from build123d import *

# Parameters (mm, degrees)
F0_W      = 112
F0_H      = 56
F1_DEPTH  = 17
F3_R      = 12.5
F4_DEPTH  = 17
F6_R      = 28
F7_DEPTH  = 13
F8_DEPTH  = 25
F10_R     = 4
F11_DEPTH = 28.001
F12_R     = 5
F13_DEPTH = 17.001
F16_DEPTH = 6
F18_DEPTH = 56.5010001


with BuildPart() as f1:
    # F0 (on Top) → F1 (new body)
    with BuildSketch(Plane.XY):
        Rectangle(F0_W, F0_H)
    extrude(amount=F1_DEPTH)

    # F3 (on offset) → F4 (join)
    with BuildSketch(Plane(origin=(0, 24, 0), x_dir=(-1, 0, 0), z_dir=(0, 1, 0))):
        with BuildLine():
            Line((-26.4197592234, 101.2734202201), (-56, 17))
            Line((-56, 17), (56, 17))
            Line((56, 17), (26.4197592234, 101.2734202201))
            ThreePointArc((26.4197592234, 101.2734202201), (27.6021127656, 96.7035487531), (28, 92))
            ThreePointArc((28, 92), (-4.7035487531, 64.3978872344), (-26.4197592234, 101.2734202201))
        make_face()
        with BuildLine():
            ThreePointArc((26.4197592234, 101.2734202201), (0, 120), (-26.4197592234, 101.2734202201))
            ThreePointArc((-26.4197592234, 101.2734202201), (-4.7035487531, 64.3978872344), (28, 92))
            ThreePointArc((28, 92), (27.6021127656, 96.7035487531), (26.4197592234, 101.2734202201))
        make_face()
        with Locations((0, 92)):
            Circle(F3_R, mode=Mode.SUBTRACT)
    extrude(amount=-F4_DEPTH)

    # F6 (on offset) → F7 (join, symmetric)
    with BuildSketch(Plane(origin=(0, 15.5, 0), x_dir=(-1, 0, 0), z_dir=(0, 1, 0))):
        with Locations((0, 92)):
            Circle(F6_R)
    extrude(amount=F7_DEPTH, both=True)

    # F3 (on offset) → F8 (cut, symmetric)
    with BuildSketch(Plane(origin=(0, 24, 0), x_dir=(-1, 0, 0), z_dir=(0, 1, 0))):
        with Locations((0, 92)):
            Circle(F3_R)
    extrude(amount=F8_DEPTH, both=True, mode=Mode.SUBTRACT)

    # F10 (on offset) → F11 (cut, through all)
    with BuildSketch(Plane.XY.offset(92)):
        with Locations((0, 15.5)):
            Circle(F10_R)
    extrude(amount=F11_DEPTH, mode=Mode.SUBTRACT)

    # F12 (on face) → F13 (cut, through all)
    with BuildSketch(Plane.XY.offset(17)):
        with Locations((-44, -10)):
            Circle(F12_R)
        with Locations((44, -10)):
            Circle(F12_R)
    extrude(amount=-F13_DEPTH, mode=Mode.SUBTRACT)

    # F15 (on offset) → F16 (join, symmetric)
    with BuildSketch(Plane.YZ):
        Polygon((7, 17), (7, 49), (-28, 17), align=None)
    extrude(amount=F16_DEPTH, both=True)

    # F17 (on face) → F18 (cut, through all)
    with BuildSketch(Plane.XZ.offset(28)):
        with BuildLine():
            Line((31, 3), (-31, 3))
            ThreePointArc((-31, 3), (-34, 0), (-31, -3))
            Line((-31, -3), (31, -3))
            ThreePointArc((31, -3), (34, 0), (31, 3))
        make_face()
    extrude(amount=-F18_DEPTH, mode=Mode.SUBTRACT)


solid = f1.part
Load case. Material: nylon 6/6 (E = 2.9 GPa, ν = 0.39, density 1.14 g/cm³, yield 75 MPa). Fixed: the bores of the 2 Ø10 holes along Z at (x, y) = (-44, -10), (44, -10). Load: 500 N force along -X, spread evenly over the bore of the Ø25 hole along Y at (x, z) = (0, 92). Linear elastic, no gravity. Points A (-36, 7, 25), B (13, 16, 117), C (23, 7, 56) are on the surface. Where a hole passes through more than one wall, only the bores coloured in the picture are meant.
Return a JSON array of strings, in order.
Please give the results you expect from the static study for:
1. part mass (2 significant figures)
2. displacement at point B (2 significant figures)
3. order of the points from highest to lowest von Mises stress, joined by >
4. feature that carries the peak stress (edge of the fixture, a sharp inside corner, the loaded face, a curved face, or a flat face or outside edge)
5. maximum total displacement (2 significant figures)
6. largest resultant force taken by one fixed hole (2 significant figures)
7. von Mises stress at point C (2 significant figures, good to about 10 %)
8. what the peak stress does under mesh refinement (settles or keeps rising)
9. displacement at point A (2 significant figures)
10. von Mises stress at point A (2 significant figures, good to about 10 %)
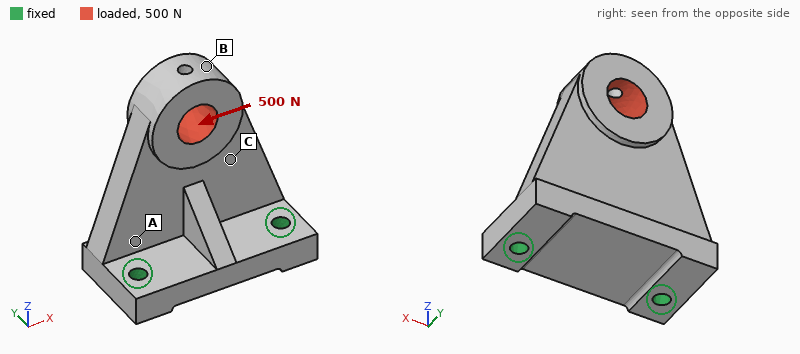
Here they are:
["270 g", "0.18 mm", "A > C > B", "edge of the fixture", "0.19 mm", "550 N", "0.94 MPa", "keeps rising", "0.044 mm", "2.1 MPa"]
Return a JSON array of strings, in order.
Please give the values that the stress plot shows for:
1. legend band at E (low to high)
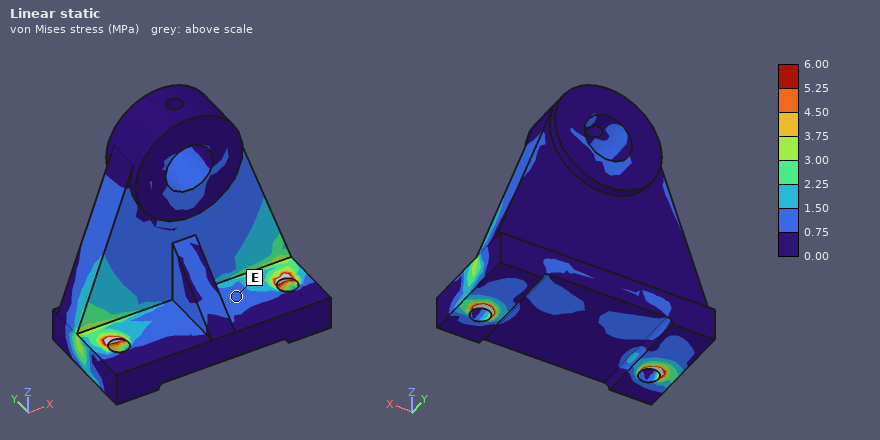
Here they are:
["0.75 to 1.50 MPa"]
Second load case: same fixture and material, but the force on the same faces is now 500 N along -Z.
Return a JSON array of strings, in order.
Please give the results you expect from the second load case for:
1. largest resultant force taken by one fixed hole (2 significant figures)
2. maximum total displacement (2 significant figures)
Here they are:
["250 N", "0.22 mm"]
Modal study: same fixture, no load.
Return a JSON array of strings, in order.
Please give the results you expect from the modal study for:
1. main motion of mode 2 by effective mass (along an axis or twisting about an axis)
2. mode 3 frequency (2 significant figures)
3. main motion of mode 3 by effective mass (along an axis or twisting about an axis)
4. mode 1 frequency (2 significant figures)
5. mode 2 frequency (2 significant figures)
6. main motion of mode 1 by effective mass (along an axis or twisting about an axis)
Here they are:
["along X", "1300 Hz", "along Z", "360 Hz", "980 Hz", "along Y"]
